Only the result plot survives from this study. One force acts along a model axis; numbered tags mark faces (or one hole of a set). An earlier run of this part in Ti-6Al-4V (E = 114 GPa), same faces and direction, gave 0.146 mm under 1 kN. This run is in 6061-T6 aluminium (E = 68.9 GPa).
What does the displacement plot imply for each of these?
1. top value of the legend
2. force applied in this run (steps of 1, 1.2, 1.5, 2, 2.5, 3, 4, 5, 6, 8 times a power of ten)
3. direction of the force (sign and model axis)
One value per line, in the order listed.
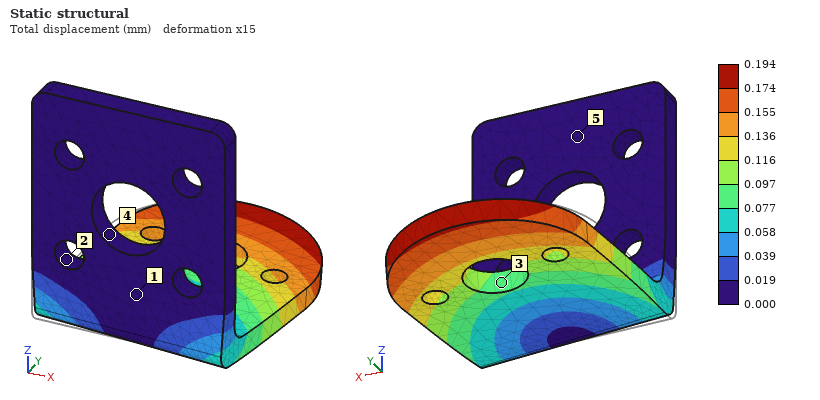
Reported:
0.194 mm
800 N
+X
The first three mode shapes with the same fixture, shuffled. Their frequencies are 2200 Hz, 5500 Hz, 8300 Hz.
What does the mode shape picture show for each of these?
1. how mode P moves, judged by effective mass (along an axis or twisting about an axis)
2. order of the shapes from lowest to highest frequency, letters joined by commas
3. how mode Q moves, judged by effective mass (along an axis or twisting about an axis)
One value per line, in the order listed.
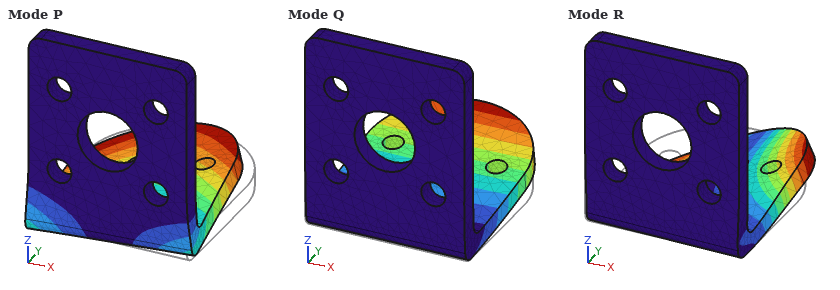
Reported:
along X
Q, P, R
along Z
